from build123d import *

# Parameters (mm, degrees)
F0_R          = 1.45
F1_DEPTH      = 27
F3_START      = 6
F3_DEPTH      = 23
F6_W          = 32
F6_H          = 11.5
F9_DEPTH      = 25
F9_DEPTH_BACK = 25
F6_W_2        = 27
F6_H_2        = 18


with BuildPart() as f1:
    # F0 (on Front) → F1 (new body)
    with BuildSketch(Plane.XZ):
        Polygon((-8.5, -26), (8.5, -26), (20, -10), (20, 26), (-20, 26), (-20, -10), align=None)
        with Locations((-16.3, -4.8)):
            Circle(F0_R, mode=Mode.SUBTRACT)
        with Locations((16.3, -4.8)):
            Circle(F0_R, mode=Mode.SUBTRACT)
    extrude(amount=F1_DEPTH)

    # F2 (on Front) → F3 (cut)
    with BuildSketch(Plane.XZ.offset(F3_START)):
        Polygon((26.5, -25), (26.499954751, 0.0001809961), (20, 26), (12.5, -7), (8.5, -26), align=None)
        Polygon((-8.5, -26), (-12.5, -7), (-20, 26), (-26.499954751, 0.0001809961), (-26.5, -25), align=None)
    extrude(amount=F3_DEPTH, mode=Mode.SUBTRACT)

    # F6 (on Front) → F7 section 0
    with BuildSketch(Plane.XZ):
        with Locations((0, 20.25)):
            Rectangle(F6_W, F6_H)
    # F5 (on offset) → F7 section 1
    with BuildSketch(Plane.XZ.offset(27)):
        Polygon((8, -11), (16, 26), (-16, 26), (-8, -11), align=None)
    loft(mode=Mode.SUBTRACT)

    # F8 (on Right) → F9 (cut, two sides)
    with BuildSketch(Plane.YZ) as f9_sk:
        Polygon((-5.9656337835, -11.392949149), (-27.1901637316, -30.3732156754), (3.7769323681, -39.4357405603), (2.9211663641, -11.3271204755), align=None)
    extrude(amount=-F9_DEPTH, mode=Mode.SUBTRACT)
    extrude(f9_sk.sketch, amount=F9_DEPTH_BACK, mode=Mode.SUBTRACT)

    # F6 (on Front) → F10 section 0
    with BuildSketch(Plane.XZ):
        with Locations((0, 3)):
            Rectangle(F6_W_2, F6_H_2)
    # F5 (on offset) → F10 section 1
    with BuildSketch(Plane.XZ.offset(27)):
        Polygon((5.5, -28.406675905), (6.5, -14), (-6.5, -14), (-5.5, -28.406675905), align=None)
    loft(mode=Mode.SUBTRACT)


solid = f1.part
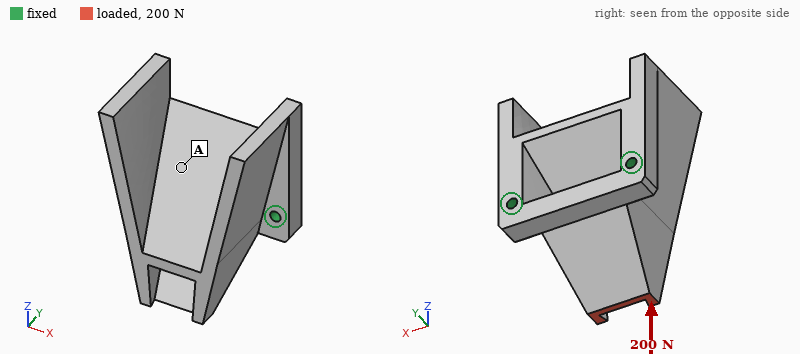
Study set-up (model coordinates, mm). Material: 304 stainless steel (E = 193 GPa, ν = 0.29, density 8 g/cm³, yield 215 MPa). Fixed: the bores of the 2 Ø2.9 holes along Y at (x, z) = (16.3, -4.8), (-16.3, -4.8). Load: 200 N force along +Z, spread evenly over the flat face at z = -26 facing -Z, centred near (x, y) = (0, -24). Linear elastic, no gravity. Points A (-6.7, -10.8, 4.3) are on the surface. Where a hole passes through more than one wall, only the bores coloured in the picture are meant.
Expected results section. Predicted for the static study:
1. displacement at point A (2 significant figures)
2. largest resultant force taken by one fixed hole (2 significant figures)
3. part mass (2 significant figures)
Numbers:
3.1 µm
100 N
88 g
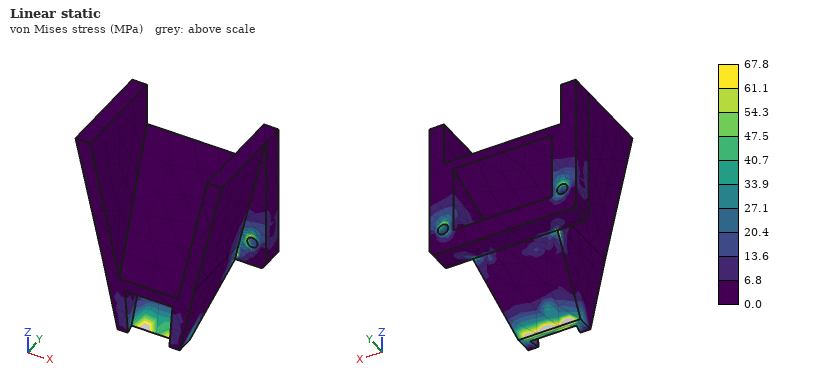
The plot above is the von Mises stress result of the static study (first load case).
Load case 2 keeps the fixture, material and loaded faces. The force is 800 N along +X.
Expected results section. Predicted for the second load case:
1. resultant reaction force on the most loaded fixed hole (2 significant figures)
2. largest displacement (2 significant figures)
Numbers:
900 N
29 µm
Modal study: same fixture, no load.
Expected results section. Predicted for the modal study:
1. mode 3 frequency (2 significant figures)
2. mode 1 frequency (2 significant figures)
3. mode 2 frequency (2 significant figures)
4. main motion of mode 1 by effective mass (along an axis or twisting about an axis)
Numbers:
4400 Hz
3100 Hz
3300 Hz
along X
